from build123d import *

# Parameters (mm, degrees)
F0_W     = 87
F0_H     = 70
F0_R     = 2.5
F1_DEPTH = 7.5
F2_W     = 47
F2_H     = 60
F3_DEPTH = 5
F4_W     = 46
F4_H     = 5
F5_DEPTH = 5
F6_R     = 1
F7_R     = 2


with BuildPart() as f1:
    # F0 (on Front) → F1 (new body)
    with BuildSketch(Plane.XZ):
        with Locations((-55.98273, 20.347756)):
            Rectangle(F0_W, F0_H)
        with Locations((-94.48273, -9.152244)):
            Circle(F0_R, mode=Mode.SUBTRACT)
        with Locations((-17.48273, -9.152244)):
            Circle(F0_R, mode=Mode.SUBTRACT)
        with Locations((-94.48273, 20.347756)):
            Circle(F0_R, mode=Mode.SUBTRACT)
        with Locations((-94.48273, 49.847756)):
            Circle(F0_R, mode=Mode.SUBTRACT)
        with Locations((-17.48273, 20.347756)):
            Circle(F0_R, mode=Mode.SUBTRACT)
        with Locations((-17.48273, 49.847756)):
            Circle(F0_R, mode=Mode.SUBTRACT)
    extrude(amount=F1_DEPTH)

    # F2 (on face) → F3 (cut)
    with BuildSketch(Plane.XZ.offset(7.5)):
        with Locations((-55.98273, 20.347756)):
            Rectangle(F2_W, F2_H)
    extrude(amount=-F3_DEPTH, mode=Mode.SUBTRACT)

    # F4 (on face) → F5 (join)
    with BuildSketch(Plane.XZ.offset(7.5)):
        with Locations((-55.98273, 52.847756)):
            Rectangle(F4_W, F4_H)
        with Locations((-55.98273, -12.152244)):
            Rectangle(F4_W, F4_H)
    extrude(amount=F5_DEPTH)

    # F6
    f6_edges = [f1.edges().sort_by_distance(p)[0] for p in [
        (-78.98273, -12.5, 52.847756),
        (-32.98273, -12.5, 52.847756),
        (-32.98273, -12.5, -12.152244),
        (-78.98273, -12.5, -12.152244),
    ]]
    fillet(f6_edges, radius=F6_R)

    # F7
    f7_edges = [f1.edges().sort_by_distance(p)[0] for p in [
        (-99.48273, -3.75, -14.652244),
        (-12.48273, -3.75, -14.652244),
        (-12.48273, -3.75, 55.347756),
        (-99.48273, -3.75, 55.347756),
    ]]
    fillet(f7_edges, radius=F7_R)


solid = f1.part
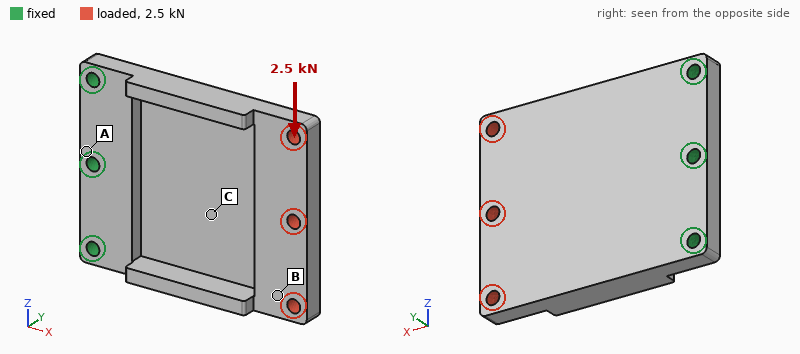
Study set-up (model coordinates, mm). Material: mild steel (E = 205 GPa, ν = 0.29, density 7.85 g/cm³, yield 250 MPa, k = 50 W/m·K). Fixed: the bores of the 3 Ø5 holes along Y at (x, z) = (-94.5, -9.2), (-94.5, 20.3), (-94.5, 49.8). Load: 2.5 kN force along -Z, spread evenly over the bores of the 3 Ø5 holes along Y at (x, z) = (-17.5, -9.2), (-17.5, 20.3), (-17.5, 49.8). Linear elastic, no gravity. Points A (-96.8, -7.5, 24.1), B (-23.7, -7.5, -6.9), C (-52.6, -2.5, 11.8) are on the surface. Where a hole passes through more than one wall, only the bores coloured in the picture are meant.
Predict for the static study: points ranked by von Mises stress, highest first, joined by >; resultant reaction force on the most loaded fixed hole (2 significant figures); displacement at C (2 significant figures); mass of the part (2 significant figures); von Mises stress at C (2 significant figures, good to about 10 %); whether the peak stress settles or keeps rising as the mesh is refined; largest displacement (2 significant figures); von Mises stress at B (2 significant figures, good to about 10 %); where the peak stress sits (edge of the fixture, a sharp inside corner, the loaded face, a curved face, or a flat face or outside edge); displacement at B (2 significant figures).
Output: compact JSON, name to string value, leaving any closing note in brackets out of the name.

{"points ranked by von Mises stress, highest first, joined by >": "C > B > A", "resultant reaction force on the most loaded fixed hole": "3.3 kN", "displacement at C": "16 µm", "mass of the part": "260 g", "von Mises stress at C": "46 MPa", "whether the peak stress settles or keeps rising as the mesh is refined": "keeps rising", "largest displacement": "77 µm", "von Mises stress at B": "33 MPa", "where the peak stress sits": "a sharp inside corner", "displacement at B": "59 µm"}
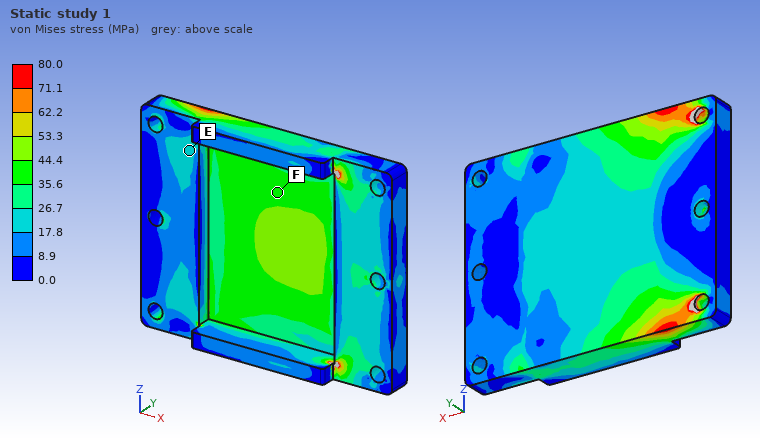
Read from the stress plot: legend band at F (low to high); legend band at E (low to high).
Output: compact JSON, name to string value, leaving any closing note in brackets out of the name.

{"legend band at F": "35.6 to 44.4 MPa", "legend band at E": "17.8 to 26.7 MPa"}
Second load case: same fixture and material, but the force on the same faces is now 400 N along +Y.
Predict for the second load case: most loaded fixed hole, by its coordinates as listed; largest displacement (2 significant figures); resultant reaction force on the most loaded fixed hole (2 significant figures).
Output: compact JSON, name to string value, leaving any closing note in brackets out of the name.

{"most loaded fixed hole, by its coordinates as listed": "(-94.5, 20.3)", "largest displacement": "0.23 mm", "resultant reaction force on the most loaded fixed hole": "1.2 kN"}
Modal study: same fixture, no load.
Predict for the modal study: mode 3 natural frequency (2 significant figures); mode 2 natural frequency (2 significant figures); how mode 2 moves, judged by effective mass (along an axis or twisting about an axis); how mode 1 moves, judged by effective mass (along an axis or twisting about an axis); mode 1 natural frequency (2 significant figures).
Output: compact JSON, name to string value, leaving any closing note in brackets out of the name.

{"mode 3 natural frequency": "5100 Hz", "mode 2 natural frequency": "1600 Hz", "how mode 2 moves, judged by effective mass": "twisting about X", "how mode 1 moves, judged by effective mass": "along Y", "mode 1 natural frequency": "770 Hz"}
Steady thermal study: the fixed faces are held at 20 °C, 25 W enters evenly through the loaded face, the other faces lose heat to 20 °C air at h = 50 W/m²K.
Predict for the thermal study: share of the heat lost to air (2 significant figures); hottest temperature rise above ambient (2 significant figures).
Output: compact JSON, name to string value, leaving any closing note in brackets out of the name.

{"share of the heat lost to air": "74 %", "hottest temperature rise above ambient": "61 K"}
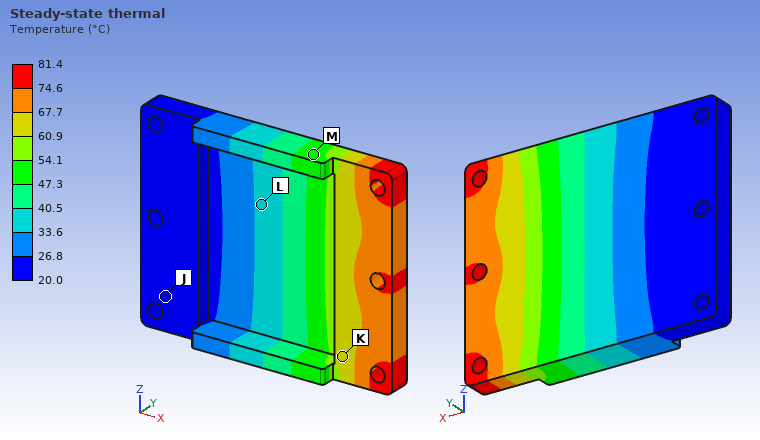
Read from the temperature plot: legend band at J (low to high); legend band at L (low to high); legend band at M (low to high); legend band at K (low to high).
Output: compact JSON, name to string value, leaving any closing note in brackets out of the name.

{"legend band at J": "20.0 to 26.8 °C", "legend band at L": "33.6 to 40.5 °C", "legend band at M": "47.3 to 54.1 °C", "legend band at K": "60.9 to 67.7 °C"}
